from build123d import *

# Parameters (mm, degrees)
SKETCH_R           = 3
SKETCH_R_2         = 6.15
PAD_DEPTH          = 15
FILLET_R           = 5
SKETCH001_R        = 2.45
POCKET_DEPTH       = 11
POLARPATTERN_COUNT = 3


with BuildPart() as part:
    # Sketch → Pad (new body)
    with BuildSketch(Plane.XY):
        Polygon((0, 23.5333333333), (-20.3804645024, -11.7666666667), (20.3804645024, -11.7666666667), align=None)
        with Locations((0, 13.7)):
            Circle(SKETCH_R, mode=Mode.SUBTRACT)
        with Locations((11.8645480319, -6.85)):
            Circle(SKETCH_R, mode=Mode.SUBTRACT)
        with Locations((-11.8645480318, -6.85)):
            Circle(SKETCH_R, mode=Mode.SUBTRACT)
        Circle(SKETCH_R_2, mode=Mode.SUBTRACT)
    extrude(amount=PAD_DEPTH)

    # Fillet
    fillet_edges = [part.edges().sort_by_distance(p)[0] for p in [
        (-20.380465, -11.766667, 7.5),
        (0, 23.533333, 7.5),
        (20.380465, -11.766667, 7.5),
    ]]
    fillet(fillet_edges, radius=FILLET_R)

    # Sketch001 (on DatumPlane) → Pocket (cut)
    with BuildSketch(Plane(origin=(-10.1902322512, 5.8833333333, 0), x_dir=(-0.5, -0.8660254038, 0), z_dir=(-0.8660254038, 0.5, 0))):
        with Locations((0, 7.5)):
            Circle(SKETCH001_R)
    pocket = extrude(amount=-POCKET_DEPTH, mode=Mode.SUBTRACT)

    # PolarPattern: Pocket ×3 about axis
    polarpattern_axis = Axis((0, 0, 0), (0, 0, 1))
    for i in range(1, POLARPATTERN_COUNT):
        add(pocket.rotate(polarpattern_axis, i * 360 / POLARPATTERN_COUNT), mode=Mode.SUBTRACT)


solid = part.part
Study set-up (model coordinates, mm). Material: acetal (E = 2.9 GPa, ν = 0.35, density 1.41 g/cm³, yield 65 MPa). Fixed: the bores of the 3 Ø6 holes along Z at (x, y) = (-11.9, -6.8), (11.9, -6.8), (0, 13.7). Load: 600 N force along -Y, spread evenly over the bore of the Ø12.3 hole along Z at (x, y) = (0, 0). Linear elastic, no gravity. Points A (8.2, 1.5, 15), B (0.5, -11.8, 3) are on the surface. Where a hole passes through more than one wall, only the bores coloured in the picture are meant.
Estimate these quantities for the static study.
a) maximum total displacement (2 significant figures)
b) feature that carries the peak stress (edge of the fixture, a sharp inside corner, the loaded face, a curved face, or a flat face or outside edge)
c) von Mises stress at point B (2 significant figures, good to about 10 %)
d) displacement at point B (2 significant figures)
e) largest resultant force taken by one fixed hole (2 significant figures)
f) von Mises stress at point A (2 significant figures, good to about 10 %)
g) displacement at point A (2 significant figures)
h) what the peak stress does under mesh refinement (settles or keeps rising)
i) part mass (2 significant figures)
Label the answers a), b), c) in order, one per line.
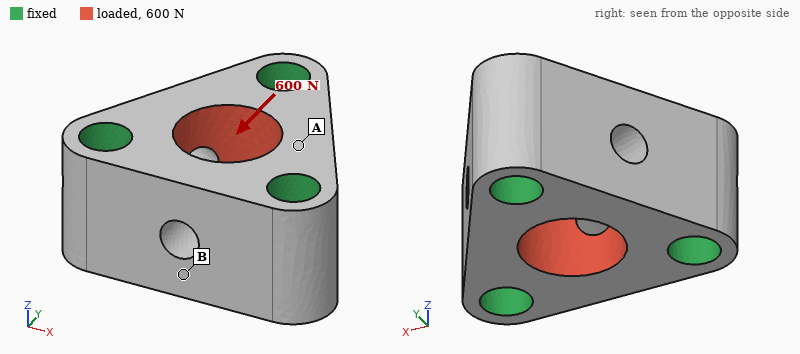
a) 12 µm
b) edge of the fixture
c) 2.4 MPa
d) 9.6 µm
e) 210 N
f) 0.61 MPa
g) 5.4 µm
h) keeps rising
i) 9.4 g
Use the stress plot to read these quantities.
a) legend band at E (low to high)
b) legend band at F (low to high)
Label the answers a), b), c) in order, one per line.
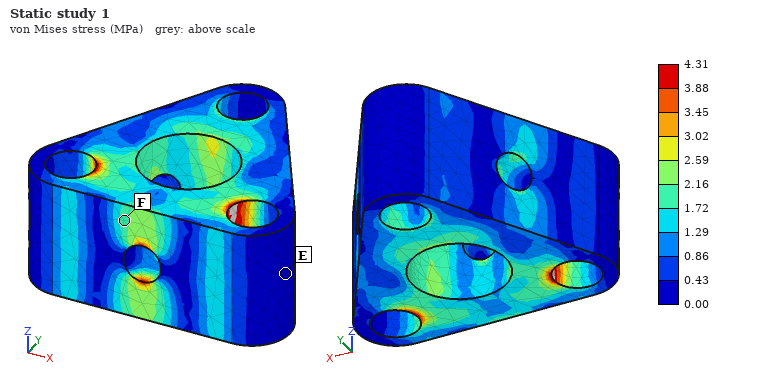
a) 0.00 to 0.43 MPa
b) 1.72 to 2.16 MPa
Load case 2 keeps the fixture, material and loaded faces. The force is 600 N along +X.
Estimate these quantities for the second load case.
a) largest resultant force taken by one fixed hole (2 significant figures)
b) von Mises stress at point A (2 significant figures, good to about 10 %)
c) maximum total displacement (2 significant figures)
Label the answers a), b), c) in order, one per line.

a) 200 N
b) 2.0 MPa
c) 11 µm
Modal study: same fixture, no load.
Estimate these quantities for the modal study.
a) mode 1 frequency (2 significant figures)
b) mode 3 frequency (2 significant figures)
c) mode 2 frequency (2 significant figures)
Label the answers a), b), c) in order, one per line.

a) 19 kHz
b) 21 kHz
c) 19 kHz
